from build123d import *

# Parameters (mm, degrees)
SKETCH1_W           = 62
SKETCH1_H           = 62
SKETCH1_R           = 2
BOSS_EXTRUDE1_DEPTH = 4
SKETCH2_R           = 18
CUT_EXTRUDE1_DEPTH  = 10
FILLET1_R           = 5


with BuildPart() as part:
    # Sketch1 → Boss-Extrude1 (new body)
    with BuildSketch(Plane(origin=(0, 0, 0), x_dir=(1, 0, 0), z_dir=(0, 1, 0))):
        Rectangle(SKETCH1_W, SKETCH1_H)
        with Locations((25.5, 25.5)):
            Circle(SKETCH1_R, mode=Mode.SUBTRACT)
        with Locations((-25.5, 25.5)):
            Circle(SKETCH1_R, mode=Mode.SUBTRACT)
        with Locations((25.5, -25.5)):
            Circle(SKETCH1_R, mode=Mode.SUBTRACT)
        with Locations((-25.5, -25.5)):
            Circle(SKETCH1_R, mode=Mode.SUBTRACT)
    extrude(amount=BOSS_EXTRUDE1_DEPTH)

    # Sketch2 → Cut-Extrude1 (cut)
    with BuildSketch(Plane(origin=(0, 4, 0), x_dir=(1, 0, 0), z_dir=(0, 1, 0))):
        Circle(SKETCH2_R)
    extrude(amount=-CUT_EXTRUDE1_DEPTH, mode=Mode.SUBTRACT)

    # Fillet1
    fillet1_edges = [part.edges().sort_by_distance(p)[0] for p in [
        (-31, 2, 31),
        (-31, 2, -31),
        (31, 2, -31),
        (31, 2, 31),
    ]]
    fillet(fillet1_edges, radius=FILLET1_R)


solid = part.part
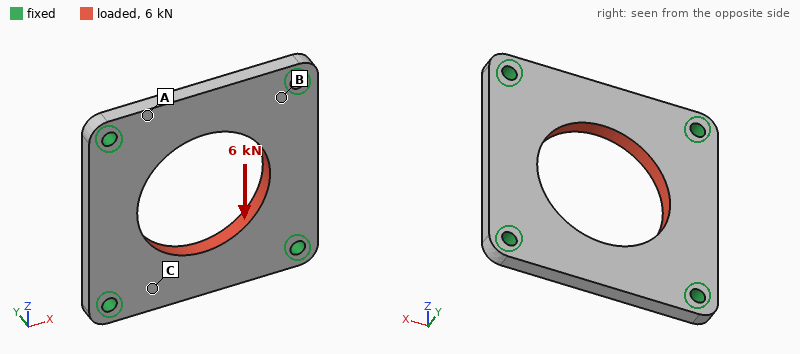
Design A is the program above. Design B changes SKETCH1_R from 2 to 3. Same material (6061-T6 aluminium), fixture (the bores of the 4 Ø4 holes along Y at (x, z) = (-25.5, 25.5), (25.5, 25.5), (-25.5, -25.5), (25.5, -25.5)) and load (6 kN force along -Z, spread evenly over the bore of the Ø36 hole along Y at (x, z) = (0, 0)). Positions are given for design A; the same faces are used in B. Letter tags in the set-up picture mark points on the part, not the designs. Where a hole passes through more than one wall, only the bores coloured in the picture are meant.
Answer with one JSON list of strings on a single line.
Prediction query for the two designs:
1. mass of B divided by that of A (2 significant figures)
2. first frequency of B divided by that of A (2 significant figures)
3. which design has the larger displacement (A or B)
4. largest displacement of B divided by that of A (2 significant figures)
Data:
["0.98", "1.1", "A", "0.89"]
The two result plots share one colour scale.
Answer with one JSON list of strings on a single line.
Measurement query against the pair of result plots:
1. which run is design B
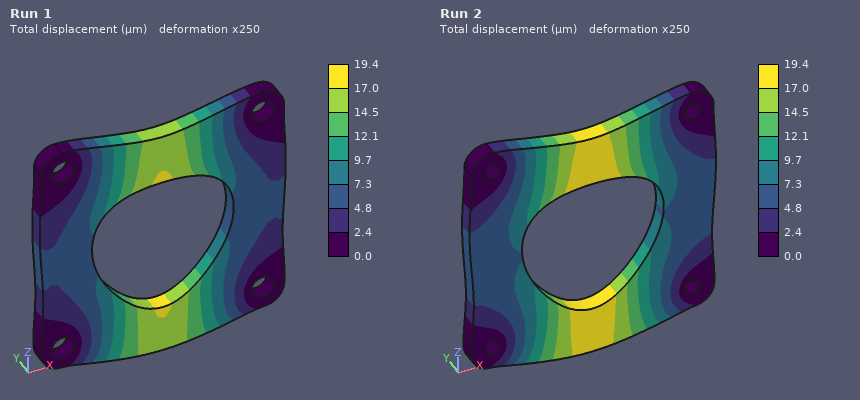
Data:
["Run 1"]
